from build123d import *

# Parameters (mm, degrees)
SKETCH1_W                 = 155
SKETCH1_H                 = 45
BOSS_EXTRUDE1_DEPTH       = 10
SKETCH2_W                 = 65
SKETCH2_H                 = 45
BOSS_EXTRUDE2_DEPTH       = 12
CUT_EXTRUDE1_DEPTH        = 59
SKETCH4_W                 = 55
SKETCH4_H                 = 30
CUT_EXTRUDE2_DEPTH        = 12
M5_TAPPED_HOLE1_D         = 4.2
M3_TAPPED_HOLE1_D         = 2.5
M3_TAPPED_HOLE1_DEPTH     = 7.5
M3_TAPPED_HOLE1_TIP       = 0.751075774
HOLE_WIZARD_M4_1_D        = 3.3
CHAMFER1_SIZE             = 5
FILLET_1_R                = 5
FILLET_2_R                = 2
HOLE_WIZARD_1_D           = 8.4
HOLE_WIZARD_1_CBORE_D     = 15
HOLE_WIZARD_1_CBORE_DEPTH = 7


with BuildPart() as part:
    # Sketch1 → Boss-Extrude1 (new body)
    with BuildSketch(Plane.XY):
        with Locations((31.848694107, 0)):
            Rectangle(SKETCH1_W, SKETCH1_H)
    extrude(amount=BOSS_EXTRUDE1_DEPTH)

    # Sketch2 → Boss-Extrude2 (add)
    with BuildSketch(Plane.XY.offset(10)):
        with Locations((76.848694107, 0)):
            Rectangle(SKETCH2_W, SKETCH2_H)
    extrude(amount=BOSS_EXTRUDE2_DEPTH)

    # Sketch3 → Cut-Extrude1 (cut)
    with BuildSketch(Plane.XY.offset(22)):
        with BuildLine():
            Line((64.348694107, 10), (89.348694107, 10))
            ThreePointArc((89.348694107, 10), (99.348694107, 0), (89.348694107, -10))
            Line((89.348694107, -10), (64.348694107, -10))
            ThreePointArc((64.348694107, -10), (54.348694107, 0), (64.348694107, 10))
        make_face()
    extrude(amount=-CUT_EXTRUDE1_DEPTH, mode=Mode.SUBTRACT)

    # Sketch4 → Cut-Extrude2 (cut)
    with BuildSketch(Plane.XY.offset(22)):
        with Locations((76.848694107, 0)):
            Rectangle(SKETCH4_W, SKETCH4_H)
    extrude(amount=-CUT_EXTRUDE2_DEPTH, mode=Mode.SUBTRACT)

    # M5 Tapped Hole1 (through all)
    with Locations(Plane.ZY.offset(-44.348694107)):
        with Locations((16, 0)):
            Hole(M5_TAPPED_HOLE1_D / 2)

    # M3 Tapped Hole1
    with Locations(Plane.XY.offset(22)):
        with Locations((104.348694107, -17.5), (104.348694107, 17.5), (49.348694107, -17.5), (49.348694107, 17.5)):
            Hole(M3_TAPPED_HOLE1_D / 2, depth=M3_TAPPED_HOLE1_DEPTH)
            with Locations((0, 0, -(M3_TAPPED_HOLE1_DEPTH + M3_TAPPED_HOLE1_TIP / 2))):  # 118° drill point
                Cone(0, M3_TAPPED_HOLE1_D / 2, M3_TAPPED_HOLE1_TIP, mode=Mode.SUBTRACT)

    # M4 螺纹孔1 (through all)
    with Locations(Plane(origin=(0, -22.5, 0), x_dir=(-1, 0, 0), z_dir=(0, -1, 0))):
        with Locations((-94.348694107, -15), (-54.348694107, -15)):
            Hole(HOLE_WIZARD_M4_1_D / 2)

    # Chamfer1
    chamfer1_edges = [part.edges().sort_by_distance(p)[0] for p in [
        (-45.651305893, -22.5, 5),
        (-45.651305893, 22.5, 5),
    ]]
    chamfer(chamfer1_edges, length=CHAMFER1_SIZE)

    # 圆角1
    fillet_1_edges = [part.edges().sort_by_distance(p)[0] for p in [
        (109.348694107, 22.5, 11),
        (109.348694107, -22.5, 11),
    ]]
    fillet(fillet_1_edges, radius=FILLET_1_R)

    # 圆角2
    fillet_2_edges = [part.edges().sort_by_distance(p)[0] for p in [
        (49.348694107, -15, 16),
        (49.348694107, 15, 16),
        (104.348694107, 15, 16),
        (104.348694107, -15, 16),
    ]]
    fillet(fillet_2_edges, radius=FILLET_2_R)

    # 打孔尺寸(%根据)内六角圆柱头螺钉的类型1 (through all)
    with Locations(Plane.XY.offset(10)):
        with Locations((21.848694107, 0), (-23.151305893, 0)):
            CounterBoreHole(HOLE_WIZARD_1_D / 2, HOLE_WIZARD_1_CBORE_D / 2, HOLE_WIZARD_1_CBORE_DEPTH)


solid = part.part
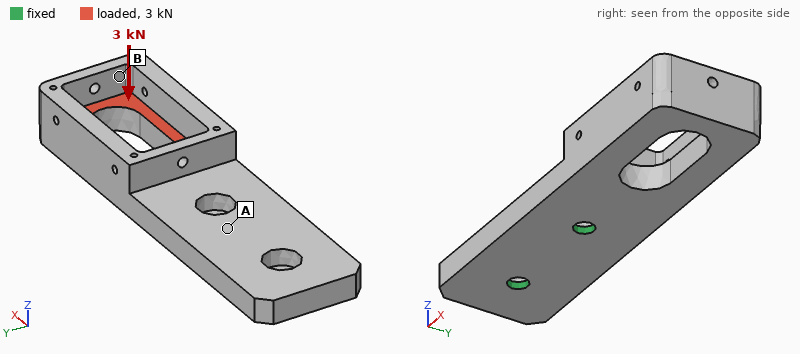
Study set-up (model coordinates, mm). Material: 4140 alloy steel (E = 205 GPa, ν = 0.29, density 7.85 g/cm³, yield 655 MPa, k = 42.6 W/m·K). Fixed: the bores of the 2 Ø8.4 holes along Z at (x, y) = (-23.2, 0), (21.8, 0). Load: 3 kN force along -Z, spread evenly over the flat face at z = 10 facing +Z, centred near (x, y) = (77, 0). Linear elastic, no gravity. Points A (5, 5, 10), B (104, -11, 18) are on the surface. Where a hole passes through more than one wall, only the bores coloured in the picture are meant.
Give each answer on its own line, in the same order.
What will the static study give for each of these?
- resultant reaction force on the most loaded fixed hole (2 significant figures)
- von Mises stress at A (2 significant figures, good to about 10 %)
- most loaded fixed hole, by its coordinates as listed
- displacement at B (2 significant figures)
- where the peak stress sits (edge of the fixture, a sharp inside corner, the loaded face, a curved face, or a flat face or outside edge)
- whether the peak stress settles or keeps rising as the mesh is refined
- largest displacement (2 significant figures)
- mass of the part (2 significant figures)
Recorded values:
9.3 kN
71 MPa
(21.8, 0)
0.54 mm
edge of the fixture
keeps rising
0.58 mm
570 g
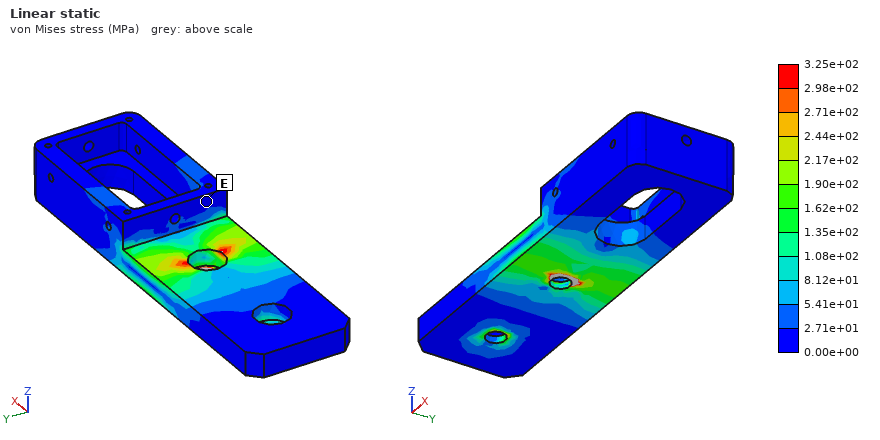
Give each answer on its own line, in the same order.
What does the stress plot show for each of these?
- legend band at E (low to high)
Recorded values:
0.00e+00 to 2.71e+01 MPa
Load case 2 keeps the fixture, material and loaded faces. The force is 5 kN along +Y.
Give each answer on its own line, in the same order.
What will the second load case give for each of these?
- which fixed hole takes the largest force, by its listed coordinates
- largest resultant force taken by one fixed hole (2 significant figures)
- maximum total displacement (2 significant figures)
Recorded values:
(21.8, 0)
10 kN
0.20 mm
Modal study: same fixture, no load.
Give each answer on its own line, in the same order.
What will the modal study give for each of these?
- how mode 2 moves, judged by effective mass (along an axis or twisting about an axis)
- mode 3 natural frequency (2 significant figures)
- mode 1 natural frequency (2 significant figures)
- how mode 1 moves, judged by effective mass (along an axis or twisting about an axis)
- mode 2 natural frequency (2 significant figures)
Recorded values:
along Y
2400 Hz
810 Hz
along Z
1700 Hz
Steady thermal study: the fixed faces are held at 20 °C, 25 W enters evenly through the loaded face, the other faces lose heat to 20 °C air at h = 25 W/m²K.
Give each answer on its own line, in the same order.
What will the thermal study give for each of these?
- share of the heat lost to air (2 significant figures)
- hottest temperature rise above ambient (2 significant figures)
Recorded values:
52 %
51 K
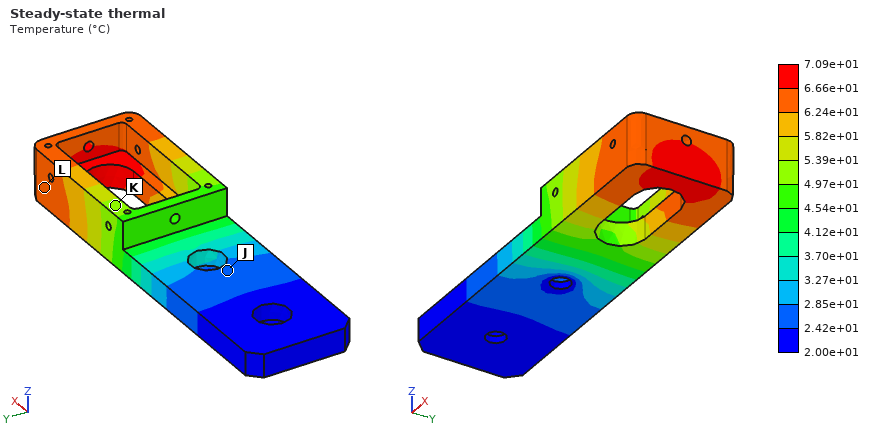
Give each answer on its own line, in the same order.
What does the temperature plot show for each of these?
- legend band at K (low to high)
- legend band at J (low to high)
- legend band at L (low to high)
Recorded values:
4.97e+01 to 5.39e+01 °C
2.42e+01 to 2.85e+01 °C
6.24e+01 to 6.66e+01 °C
